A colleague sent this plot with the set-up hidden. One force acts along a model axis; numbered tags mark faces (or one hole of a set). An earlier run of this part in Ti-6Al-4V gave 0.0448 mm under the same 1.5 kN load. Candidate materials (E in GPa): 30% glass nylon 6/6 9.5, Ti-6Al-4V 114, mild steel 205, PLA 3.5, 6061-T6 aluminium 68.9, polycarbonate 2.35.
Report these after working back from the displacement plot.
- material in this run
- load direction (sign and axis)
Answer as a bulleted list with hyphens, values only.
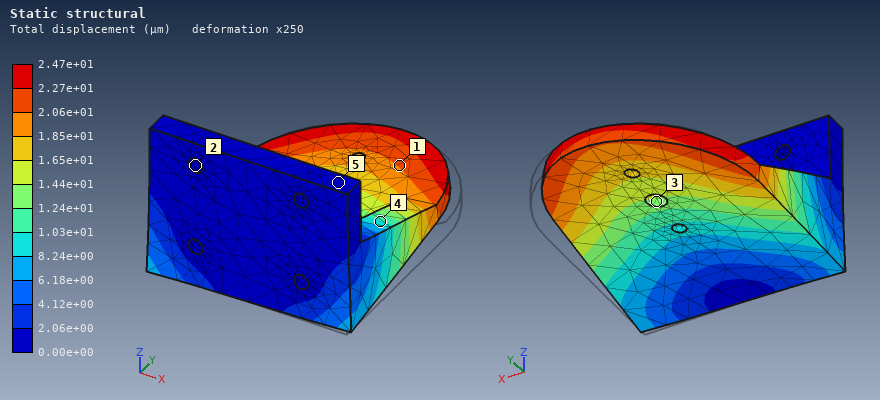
- mild steel
- -X
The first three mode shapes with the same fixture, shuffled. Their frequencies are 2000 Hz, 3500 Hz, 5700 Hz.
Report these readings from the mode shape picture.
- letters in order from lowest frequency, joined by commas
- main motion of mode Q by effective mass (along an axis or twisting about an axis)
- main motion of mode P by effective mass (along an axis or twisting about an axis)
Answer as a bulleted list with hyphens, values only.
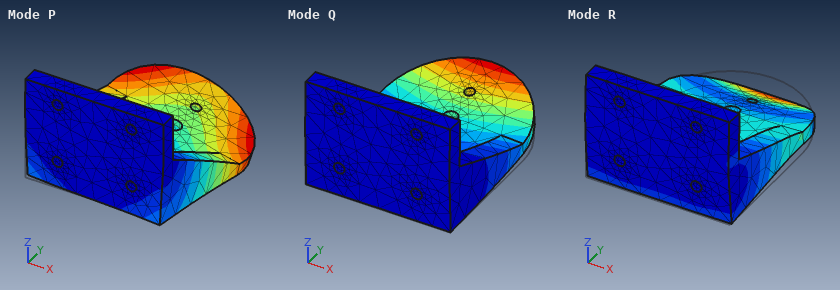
- Q, P, R
- along Z
- along X
